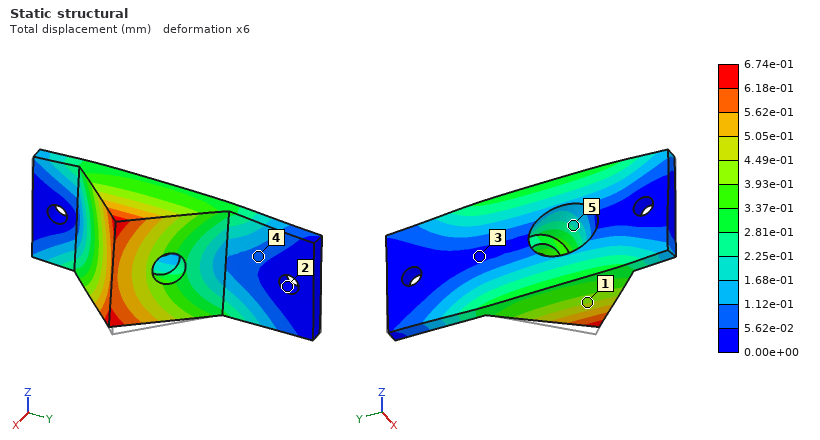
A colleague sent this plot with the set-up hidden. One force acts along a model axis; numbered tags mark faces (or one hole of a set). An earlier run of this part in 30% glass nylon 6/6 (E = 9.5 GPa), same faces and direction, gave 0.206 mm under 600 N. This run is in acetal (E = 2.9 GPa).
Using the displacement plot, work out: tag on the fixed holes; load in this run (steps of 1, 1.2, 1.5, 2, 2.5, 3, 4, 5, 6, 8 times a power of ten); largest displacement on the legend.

2
600 N
6.74e-01 mm
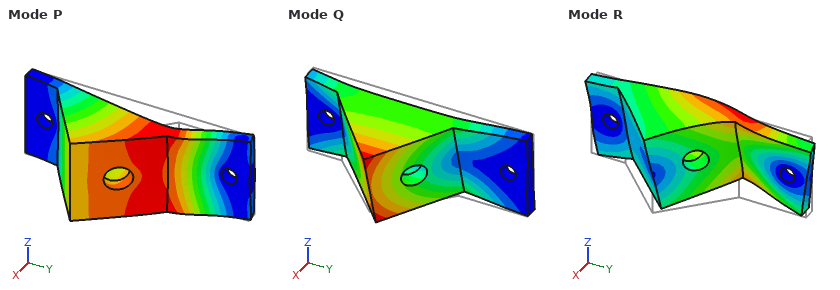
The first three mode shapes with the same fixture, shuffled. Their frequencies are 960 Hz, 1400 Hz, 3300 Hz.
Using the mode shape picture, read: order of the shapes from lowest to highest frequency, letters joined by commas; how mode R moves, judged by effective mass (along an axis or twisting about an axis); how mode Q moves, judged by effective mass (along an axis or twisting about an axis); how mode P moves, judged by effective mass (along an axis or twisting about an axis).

Q, P, R
along Z
along Z
along X
